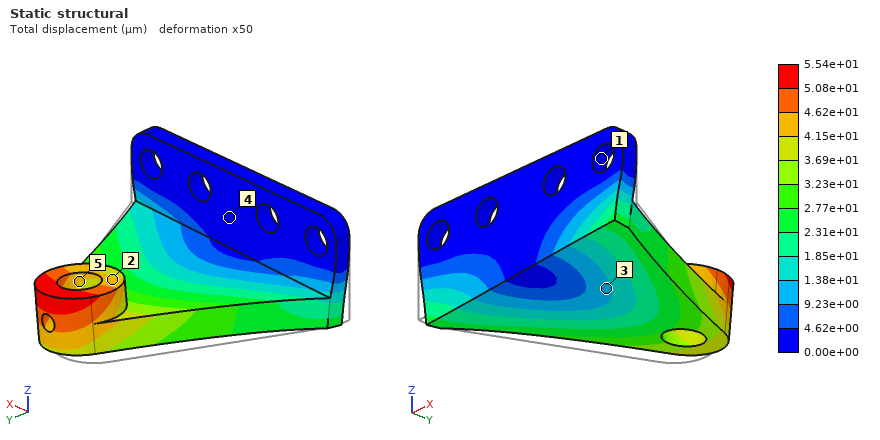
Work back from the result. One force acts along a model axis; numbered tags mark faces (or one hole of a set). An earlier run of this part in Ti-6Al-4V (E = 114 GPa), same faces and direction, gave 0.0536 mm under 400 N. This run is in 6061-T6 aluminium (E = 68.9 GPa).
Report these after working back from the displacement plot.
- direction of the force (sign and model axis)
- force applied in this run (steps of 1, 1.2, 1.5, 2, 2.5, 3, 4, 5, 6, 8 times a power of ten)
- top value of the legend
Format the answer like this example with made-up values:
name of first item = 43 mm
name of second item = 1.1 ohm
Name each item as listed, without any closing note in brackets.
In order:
direction of the force = +X
force applied in this run = 250 N
top value of the legend = 5.54e+01 µm
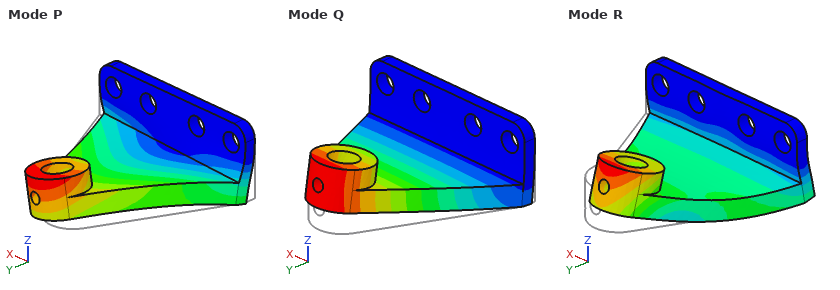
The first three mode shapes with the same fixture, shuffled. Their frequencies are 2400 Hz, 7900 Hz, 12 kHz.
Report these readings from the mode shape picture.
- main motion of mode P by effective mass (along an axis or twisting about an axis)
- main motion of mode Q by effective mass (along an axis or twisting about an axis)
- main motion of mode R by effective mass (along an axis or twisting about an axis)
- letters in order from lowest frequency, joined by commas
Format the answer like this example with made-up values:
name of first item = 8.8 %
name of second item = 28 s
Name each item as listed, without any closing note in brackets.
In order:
main motion of mode P by effective mass = along X
main motion of mode Q by effective mass = along Z
main motion of mode R by effective mass = along Y
letters in order from lowest frequency, joined by commas = Q, P, R
